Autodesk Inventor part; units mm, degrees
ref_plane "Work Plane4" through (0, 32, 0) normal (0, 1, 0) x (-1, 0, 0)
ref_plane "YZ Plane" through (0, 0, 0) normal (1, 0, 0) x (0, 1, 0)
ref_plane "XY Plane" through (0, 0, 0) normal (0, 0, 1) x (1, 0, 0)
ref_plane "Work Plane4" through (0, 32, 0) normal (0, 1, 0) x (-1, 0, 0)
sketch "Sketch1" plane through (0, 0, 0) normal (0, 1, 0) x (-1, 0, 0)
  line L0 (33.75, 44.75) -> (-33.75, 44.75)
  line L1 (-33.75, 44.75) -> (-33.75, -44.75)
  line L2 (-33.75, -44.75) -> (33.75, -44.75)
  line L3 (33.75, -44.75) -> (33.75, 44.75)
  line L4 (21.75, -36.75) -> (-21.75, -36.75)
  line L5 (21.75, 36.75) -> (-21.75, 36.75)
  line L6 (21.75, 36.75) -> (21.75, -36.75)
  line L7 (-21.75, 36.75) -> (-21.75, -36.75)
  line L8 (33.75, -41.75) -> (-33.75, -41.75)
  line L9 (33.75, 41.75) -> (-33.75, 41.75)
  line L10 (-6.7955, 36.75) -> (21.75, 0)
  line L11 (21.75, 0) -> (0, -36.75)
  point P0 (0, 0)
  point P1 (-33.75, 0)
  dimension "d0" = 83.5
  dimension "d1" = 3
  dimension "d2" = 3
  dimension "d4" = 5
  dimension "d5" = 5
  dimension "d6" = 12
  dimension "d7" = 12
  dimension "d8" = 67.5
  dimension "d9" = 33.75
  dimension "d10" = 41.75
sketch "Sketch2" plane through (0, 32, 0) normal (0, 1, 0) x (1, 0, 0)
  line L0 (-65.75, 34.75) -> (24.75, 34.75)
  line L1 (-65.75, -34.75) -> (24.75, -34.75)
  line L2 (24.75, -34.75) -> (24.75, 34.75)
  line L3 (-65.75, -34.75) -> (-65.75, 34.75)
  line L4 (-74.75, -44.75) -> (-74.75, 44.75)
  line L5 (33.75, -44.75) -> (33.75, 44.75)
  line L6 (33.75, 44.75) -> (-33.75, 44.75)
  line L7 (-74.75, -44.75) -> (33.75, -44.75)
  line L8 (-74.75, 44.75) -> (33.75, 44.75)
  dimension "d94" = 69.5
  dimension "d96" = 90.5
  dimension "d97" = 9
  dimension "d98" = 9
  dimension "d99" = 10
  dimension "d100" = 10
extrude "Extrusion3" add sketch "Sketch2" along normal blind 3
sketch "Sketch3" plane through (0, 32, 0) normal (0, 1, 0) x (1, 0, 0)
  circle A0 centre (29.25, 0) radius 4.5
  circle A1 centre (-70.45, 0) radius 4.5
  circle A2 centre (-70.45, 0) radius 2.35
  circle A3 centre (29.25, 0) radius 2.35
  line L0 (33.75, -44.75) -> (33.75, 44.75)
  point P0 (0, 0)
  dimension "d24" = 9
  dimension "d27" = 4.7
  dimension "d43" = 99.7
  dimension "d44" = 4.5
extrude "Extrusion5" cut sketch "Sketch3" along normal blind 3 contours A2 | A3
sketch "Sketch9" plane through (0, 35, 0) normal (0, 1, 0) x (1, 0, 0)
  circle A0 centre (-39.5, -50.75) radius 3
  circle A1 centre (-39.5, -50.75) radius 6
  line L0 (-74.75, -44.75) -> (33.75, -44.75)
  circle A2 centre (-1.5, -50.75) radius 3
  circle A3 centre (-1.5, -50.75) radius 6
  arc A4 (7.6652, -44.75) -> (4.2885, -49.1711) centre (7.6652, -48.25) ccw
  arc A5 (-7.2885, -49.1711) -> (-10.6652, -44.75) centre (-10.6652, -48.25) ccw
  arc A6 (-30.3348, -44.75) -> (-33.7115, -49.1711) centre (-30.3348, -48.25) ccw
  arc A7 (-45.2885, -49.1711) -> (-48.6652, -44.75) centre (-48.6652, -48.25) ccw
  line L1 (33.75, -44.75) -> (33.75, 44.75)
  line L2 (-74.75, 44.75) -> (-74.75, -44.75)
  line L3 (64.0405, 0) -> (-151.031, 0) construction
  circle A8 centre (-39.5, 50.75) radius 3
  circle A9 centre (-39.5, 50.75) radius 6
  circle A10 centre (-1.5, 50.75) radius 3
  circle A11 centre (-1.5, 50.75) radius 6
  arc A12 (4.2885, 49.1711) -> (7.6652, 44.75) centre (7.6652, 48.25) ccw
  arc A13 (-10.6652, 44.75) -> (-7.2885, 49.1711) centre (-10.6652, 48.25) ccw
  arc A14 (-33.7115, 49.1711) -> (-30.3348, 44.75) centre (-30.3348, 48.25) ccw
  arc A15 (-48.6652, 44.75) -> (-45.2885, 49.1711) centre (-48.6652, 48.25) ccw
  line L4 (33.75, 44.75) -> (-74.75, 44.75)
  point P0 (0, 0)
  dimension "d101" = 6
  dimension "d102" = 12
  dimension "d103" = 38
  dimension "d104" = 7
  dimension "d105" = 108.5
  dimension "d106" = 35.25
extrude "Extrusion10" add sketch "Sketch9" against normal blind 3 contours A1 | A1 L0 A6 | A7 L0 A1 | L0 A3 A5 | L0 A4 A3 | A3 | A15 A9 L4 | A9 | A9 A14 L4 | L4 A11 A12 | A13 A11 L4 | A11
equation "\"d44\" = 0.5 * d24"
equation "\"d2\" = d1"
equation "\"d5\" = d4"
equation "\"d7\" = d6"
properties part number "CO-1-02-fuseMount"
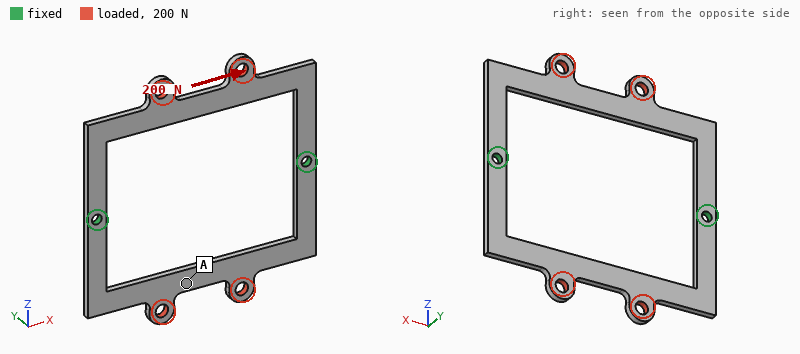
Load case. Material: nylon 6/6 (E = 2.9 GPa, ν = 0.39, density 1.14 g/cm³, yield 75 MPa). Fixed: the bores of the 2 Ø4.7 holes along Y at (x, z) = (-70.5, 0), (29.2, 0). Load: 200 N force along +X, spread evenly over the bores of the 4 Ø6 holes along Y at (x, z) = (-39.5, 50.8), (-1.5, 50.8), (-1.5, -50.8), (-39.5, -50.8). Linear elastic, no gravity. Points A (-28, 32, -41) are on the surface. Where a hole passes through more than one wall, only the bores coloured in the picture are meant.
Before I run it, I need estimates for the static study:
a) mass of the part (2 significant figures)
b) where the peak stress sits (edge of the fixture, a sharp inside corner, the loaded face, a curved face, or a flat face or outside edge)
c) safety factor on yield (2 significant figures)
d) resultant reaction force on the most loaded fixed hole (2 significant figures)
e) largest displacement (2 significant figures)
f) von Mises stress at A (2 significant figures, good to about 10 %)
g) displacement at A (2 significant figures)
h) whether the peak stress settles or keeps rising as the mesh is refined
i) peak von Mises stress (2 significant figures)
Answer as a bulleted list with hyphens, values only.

- 13 g
- a flat face or outside edge
- 2.9
- 100 N
- 0.82 mm
- 2.6 MPa
- 0.76 mm
- settles
- 26 MPa
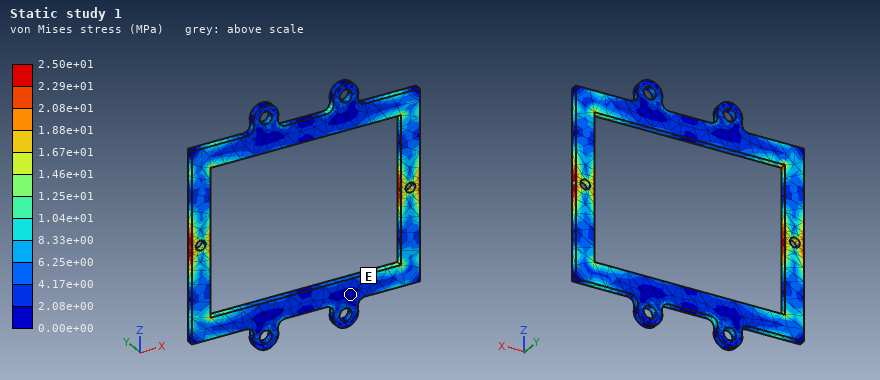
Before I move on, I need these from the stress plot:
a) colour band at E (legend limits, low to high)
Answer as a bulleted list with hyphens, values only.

- 0.00e+00 to 2.08e+00 MPa
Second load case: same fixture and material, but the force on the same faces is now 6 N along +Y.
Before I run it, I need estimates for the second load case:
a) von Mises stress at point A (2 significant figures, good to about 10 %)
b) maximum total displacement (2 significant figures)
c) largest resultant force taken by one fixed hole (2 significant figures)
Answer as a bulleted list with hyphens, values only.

- 1.8 MPa
- 1.6 mm
- 3.0 N
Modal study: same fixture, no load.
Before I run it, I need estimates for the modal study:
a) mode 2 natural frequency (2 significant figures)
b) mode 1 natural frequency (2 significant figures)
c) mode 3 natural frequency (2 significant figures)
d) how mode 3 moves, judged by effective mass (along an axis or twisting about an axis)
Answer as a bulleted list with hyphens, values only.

- 150 Hz
- 150 Hz
- 350 Hz
- twisting about Z
